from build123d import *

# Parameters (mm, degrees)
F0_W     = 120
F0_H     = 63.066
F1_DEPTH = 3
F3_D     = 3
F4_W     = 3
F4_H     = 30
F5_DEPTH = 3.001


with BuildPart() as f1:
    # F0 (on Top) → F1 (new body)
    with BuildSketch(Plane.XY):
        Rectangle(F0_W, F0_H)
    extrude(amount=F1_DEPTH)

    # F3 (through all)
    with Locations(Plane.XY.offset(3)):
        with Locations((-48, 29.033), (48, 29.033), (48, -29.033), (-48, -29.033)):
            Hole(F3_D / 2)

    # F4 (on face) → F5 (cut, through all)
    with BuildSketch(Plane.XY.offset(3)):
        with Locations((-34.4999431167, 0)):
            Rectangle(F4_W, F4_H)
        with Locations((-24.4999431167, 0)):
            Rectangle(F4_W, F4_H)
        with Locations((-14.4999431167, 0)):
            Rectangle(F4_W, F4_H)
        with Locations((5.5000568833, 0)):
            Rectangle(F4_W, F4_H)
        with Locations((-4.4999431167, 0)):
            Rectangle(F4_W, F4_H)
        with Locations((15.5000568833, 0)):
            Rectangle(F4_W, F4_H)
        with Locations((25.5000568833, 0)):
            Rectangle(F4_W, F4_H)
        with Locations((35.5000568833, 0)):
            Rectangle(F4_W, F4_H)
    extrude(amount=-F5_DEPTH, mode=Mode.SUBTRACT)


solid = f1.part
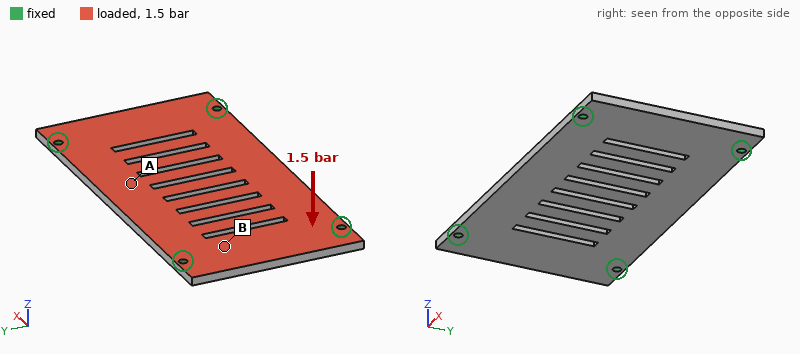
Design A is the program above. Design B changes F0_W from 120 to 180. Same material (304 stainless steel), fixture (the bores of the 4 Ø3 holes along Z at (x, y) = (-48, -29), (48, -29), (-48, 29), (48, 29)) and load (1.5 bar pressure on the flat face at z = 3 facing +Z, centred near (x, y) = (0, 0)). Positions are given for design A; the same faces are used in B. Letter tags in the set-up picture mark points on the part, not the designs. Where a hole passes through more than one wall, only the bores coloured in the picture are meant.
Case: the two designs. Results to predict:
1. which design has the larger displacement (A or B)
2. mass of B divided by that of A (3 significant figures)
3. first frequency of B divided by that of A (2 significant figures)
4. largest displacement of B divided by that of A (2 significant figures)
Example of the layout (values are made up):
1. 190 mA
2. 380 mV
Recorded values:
1. B
2. 1.55
3. 0.79
4. 1.2
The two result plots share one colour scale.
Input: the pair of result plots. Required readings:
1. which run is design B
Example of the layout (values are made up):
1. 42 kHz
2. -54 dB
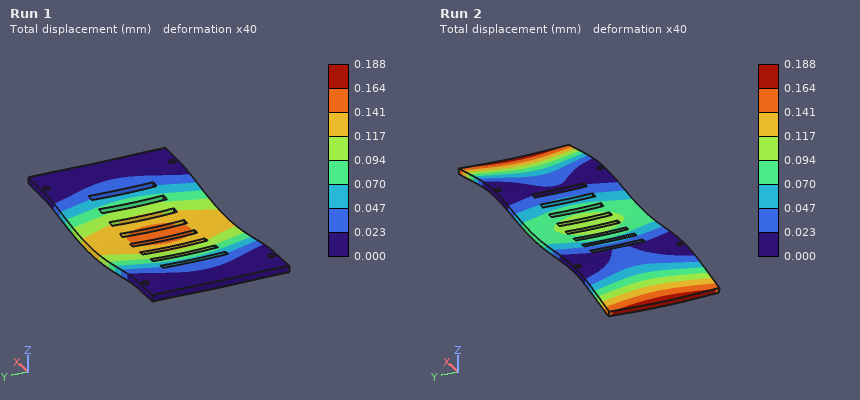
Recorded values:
1. Run 2
